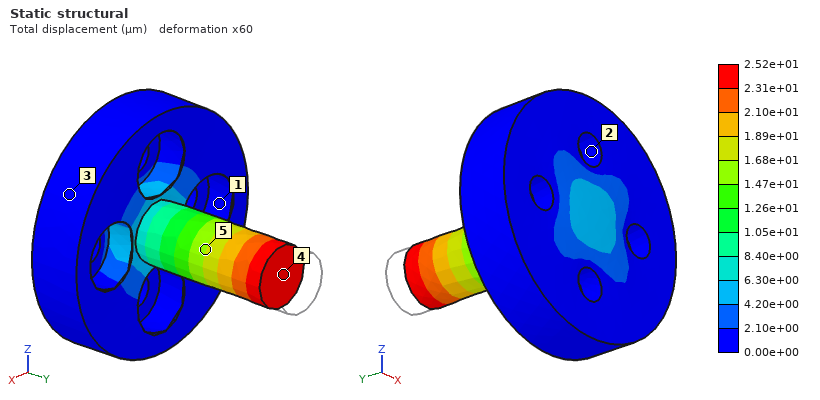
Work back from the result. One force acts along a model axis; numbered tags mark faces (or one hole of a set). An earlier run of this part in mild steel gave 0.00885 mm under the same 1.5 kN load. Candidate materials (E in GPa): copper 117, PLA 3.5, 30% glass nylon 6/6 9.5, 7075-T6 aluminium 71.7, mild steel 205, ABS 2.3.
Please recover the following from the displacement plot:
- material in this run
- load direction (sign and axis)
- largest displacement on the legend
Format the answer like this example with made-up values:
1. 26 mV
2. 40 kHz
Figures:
1. 7075-T6 aluminium
2. -Y
3. 2.52e+01 µm
